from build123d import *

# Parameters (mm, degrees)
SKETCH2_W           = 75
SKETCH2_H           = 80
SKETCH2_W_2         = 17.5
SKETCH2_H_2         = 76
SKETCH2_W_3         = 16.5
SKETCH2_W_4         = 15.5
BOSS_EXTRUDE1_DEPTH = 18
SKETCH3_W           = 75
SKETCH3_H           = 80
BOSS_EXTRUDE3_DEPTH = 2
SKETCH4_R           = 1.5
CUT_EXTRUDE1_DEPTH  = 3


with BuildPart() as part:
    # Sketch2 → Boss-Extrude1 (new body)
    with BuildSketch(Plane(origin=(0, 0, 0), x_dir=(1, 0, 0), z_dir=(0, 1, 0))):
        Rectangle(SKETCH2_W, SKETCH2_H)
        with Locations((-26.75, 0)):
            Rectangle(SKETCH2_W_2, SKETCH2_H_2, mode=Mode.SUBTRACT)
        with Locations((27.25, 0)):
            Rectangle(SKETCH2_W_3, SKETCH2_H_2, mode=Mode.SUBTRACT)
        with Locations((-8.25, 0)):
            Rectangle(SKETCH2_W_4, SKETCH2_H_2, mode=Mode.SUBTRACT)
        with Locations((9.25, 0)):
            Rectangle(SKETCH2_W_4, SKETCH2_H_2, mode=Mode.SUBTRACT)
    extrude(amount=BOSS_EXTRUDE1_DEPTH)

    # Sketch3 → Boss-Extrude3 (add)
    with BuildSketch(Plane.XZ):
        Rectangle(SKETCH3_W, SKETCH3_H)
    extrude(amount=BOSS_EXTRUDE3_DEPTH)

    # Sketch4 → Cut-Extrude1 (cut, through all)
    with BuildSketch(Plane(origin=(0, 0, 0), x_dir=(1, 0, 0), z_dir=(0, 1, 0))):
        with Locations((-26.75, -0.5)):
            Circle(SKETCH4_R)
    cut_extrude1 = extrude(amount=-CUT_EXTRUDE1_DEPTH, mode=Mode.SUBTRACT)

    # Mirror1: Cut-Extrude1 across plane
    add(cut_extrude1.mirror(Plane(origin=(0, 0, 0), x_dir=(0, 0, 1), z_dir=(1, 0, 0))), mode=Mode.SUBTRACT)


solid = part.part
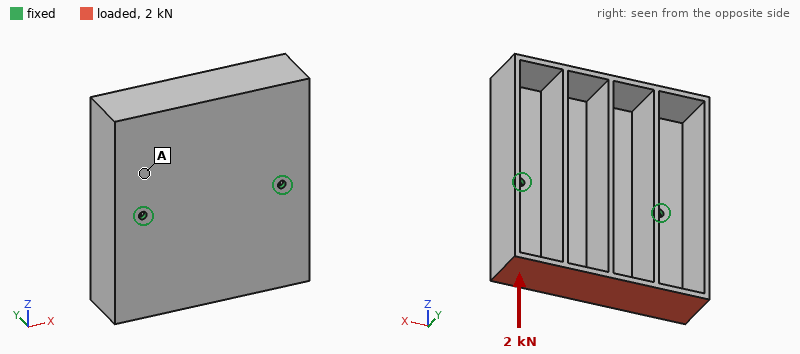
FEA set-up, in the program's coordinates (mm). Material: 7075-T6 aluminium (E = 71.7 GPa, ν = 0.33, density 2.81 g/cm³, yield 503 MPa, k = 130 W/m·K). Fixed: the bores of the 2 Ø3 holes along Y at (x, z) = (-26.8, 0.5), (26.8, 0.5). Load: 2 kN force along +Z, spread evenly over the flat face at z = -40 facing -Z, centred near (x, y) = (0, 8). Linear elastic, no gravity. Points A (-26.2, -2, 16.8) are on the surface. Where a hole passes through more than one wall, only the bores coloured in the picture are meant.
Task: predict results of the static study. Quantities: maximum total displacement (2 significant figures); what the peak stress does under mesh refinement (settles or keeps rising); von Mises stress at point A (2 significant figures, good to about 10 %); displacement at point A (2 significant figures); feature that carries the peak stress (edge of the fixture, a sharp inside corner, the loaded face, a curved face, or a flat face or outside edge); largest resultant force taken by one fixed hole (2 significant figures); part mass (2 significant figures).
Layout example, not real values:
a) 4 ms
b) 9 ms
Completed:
a) 1.0 mm
b) keeps rising
c) 40 MPa
d) 0.35 mm
e) edge of the fixture
f) 1.0 kN
g) 87 g
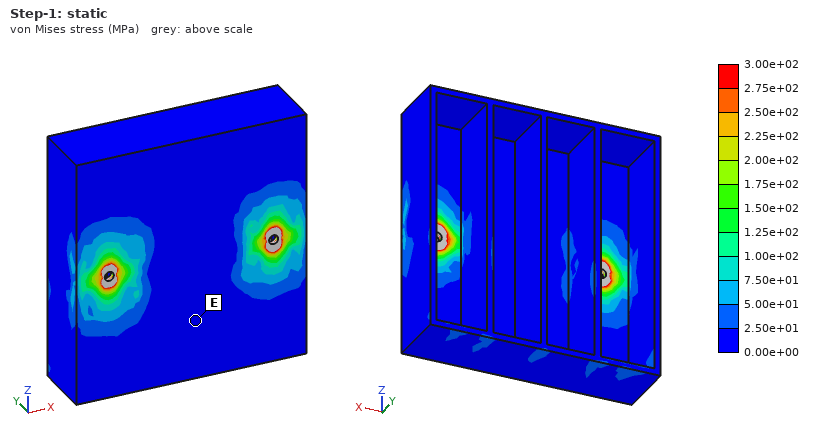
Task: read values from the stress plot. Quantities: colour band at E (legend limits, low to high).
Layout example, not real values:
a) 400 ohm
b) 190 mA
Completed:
a) 0.00e+00 to 2.50e+01 MPa
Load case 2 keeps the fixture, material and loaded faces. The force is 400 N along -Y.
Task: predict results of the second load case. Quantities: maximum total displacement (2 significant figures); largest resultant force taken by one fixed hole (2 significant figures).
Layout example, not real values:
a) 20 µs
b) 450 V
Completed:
a) 0.94 mm
b) 200 N
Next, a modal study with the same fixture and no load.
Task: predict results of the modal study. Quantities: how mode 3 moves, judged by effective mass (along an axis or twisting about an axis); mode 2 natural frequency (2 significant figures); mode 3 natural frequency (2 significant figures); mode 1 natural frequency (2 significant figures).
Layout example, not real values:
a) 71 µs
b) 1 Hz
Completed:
a) along Y
b) 1200 Hz
c) 2500 Hz
d) 550 Hz
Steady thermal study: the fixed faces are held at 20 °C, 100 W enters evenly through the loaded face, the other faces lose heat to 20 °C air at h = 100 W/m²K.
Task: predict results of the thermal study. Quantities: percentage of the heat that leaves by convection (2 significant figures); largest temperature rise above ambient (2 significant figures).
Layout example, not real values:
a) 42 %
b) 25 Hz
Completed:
a) 75 %
b) 82 K
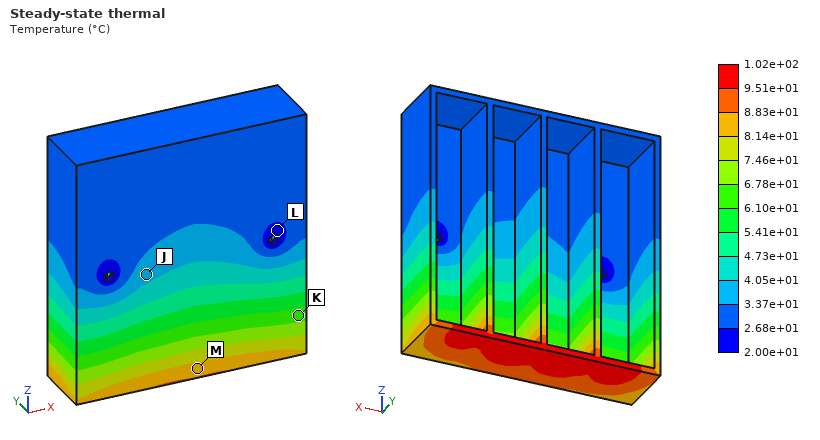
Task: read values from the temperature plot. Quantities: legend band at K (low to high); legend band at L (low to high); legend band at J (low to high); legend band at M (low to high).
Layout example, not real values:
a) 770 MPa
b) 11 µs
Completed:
a) 6.10e+01 to 6.78e+01 °C
b) 2.00e+01 to 2.68e+01 °C
c) 3.37e+01 to 4.05e+01 °C
d) 8.14e+01 to 8.83e+01 °C
